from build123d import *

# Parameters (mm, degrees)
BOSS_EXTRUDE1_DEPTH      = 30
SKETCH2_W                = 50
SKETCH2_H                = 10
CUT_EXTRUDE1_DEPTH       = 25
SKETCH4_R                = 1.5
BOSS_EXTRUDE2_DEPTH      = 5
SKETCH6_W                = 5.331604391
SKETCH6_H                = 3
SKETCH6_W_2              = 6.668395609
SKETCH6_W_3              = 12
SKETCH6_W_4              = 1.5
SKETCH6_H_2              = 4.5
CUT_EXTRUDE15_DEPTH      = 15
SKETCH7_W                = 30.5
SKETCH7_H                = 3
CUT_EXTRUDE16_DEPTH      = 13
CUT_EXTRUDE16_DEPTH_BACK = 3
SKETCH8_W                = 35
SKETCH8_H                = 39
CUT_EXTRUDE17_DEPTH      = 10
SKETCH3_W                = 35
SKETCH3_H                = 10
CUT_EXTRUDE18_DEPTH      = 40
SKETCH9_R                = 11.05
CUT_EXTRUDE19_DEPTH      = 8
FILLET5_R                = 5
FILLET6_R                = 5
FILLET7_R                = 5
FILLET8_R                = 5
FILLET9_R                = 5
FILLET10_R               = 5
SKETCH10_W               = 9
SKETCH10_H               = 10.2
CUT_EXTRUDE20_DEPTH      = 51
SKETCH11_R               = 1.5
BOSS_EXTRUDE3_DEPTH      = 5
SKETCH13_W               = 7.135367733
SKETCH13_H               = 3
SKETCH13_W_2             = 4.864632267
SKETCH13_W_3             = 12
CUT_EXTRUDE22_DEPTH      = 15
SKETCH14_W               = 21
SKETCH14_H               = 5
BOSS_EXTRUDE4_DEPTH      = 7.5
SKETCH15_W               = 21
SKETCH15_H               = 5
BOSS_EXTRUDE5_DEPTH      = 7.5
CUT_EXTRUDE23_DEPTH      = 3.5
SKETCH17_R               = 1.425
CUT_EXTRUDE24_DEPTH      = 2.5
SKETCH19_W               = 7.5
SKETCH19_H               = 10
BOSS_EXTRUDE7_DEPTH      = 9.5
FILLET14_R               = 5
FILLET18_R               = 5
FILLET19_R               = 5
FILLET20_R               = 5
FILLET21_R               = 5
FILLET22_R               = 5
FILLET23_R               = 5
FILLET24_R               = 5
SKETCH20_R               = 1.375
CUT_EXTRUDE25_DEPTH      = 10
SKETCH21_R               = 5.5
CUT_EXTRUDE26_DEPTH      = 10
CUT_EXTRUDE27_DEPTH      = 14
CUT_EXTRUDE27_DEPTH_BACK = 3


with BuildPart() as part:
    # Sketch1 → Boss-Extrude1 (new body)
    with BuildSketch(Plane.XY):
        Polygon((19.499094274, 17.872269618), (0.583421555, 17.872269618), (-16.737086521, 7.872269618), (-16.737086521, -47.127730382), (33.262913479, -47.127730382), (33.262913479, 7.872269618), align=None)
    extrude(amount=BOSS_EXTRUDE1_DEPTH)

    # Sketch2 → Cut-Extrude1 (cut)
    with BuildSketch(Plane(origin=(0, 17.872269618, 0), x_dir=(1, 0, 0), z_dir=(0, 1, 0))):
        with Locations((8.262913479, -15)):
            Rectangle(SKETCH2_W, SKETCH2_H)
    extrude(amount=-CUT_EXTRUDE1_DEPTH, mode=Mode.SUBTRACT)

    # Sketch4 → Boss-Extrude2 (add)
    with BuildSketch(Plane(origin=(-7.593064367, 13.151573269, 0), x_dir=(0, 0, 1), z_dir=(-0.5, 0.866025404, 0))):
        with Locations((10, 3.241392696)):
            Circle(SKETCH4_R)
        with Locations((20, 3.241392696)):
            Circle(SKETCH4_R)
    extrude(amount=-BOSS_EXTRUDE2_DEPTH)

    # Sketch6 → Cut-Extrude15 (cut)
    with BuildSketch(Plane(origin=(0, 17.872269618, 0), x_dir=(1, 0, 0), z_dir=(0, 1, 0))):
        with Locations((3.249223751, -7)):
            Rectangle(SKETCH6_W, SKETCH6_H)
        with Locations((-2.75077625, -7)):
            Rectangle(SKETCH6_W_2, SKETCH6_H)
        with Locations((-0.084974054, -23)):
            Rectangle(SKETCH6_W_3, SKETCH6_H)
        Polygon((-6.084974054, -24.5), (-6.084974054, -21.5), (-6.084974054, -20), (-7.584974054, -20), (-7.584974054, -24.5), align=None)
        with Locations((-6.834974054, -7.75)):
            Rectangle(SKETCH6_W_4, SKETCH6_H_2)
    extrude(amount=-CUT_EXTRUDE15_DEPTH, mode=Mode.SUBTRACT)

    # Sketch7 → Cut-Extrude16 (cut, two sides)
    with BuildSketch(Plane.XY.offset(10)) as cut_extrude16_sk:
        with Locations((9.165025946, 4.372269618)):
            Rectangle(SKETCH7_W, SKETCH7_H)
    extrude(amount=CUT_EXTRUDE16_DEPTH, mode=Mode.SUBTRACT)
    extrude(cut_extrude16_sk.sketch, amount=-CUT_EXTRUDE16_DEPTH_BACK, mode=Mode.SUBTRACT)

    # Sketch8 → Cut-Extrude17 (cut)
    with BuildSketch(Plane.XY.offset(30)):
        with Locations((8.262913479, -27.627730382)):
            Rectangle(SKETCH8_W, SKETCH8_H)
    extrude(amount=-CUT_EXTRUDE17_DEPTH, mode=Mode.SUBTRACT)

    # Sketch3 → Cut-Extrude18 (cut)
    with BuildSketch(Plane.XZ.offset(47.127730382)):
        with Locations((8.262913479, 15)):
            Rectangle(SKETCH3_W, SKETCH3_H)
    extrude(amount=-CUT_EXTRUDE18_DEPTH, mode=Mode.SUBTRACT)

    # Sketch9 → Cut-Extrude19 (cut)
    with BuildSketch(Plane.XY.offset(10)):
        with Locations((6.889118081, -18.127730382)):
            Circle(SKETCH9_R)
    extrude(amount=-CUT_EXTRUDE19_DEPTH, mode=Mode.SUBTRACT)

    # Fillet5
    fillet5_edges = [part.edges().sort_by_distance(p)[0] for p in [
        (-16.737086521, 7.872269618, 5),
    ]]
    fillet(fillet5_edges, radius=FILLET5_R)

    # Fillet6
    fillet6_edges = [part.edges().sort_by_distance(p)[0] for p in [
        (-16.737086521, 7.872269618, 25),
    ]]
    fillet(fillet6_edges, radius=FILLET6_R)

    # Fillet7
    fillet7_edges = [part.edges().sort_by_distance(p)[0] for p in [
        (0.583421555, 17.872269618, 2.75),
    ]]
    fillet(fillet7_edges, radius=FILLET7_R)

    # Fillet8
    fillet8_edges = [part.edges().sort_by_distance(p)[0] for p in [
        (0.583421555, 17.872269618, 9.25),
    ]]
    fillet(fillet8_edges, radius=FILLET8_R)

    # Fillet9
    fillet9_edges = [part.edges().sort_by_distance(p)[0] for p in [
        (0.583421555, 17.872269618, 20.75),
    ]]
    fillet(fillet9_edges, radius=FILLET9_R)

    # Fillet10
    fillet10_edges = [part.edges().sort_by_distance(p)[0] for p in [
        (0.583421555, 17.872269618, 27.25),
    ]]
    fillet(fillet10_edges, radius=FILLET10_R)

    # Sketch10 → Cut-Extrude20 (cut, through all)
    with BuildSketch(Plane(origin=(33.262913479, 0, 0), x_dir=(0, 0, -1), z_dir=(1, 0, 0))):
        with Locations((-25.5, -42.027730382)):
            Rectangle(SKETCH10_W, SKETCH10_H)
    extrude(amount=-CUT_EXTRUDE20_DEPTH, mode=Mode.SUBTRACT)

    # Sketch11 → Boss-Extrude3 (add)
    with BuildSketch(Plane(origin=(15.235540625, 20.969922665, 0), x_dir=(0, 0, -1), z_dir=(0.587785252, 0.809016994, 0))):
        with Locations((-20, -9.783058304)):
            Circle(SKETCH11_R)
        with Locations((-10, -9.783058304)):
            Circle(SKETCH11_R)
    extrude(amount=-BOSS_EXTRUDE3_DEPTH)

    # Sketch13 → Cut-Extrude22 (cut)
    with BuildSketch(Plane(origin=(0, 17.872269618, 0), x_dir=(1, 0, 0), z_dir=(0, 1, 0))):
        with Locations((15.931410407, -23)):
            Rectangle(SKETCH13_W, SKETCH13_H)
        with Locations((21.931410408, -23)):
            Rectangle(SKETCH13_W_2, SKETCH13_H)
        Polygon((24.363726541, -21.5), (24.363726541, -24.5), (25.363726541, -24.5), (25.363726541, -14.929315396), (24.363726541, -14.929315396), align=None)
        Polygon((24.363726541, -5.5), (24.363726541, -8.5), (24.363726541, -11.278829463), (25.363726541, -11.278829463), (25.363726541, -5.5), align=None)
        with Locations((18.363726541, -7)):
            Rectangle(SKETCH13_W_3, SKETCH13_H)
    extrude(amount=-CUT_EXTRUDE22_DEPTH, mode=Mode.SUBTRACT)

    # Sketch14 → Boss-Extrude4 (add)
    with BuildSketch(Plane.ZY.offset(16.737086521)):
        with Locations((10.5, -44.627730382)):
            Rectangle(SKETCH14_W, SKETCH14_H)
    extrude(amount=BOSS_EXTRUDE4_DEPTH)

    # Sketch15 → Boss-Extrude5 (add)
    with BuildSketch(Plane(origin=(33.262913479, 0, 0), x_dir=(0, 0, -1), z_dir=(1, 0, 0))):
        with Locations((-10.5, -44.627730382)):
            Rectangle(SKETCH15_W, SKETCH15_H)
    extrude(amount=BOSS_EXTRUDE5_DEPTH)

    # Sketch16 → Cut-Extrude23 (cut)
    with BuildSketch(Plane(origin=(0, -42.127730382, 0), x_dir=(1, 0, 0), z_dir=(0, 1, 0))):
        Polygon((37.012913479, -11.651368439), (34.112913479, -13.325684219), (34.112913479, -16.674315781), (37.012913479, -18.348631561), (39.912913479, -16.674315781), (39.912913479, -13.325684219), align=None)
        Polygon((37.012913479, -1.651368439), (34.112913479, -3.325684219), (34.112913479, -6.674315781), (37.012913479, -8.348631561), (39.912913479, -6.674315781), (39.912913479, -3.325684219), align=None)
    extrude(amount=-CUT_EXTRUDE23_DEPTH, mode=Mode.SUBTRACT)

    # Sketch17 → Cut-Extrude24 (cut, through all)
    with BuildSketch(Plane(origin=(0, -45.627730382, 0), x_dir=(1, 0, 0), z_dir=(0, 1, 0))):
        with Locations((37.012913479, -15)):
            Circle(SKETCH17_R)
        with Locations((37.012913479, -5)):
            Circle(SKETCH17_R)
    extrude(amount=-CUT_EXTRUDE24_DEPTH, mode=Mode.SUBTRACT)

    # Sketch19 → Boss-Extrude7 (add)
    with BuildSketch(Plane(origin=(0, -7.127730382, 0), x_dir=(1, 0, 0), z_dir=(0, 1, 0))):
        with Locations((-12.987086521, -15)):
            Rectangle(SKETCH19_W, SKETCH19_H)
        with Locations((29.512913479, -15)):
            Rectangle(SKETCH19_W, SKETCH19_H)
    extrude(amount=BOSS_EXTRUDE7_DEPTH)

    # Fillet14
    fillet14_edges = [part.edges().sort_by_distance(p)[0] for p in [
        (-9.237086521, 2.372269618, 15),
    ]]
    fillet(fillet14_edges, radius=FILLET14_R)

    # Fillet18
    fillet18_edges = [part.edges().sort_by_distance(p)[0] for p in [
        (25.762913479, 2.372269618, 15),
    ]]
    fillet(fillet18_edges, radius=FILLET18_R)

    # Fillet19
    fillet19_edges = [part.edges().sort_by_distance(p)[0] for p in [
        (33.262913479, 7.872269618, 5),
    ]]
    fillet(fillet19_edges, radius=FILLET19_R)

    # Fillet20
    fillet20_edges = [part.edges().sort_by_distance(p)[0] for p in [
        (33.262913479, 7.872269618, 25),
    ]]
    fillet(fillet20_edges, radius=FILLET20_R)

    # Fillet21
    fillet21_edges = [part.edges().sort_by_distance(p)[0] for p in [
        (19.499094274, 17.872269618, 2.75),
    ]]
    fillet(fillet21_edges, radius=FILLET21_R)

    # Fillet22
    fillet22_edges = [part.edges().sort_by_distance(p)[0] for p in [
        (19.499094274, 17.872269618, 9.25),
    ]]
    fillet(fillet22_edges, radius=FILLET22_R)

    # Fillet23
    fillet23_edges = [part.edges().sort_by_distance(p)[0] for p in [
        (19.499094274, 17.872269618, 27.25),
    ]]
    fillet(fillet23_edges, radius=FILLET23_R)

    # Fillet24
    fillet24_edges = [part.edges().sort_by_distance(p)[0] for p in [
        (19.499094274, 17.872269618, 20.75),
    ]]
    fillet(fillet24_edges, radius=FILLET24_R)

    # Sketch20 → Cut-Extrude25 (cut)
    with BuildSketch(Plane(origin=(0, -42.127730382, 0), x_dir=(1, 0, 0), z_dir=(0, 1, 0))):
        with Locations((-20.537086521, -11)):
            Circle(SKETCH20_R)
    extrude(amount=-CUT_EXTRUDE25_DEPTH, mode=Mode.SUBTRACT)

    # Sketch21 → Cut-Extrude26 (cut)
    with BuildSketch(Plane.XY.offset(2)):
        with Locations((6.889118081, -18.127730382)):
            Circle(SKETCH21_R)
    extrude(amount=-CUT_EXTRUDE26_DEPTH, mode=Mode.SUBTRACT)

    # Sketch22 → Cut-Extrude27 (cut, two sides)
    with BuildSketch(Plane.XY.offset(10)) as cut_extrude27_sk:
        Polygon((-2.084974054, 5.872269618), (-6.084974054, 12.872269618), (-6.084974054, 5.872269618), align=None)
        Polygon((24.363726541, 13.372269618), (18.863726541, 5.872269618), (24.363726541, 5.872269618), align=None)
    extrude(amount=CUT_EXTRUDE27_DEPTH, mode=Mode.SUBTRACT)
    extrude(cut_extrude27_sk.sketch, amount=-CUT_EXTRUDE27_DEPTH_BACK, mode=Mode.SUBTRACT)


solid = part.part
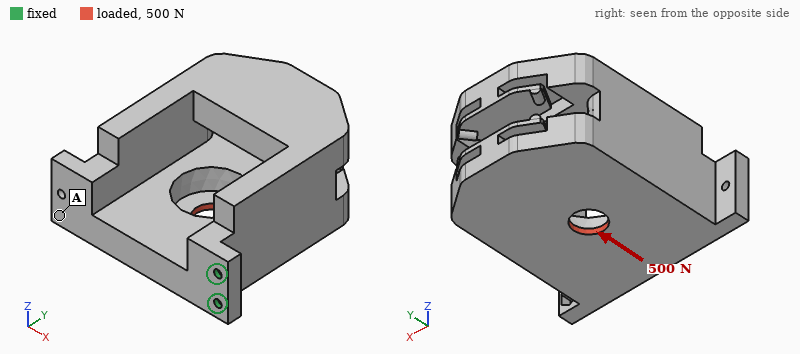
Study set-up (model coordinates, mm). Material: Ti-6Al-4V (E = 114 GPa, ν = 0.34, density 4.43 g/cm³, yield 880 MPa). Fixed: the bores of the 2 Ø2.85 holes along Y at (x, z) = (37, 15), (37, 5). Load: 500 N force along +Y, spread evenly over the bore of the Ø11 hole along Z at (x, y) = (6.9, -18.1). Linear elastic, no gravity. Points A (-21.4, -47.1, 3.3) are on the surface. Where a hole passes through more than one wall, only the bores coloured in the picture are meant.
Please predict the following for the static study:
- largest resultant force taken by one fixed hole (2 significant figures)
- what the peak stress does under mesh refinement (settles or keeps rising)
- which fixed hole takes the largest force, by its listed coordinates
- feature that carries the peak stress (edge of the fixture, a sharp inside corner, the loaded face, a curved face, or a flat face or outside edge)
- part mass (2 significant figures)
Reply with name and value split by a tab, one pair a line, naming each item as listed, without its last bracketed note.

largest resultant force taken by one fixed hole	680 N
what the peak stress does under mesh refinement	keeps rising
which fixed hole takes the largest force, by its listed coordinates	(37, 5)
feature that carries the peak stress	edge of the fixture
part mass	220 g
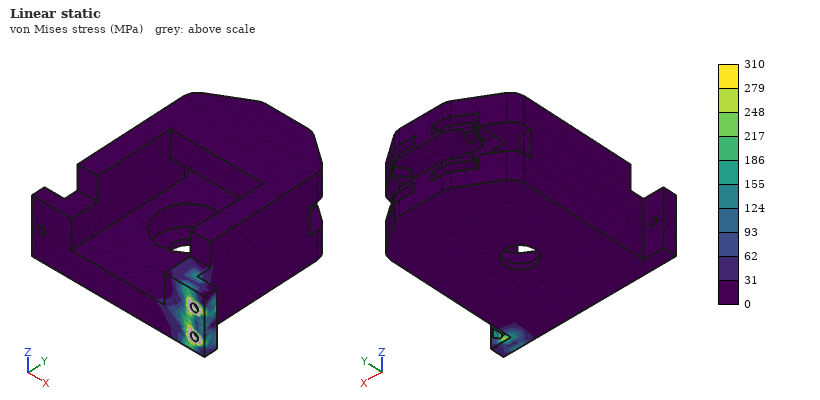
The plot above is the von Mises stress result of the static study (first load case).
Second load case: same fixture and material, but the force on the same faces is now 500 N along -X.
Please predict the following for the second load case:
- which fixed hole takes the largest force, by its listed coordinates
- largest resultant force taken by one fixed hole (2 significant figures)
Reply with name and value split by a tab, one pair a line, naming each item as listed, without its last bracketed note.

which fixed hole takes the largest force, by its listed coordinates	(37, 5)
largest resultant force taken by one fixed hole	650 N
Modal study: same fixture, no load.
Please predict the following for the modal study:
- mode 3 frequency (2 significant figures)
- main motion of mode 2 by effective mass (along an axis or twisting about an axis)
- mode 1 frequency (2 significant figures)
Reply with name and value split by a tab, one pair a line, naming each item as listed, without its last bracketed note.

mode 3 frequency	1200 Hz
main motion of mode 2 by effective mass	along Z
mode 1 frequency	220 Hz
